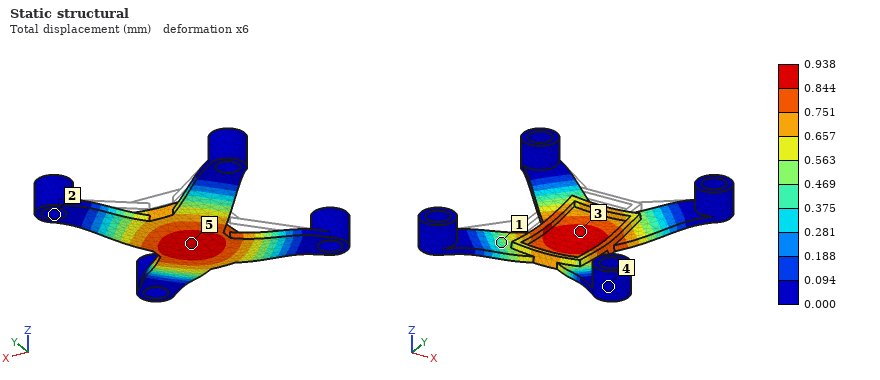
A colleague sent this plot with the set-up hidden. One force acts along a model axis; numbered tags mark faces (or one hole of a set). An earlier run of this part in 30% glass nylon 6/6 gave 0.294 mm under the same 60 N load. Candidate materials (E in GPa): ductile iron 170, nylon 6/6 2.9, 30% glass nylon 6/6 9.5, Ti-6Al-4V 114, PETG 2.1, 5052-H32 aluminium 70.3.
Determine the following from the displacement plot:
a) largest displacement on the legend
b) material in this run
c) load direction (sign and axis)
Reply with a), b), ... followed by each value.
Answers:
a) 0.938 mm
b) nylon 6/6
c) -Z
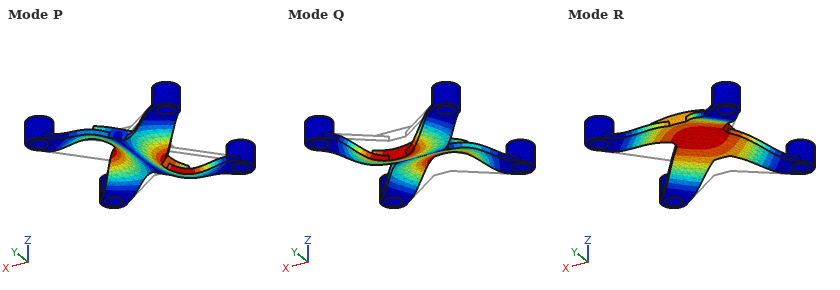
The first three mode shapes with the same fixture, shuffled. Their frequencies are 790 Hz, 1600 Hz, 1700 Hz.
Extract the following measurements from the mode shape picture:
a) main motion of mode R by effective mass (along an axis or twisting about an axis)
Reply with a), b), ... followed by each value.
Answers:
a) along Z
